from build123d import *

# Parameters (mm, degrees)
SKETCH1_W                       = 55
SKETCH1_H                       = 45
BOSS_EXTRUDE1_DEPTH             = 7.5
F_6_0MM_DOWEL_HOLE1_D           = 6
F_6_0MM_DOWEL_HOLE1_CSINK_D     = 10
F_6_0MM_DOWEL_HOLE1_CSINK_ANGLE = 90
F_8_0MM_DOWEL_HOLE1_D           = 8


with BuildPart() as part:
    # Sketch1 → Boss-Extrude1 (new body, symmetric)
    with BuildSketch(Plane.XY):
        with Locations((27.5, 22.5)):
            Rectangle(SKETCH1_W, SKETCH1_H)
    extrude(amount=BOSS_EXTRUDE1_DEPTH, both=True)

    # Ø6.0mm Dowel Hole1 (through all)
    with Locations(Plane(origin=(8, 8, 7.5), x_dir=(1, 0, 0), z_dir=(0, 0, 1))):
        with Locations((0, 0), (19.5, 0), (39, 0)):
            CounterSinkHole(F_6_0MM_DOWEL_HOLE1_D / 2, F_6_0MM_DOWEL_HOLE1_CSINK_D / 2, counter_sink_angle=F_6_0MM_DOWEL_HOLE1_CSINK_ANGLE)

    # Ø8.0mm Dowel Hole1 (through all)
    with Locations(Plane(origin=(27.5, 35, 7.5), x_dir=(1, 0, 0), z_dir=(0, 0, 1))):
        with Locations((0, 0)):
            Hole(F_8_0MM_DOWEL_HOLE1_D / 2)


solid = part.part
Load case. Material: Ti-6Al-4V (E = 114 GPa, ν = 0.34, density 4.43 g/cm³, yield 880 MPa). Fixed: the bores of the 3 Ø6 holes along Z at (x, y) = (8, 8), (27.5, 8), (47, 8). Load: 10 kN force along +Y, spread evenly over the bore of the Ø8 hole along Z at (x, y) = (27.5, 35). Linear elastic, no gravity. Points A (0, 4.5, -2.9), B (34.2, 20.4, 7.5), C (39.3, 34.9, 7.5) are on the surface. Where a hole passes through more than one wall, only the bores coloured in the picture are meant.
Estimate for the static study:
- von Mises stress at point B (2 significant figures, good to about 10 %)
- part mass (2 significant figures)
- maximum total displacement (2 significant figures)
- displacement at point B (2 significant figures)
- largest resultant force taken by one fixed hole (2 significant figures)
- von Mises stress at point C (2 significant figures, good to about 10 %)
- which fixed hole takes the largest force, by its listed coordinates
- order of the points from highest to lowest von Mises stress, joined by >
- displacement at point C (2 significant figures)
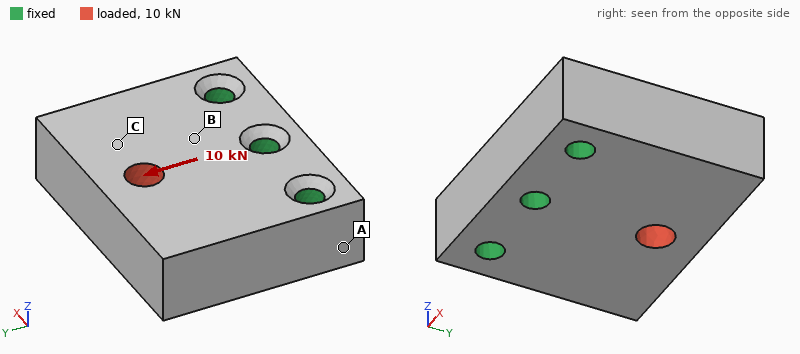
19 MPa
150 g
8.4 µm
2.4 µm
4.3 kN
11 MPa
(27.5, 8)
B > C > A
3.4 µm
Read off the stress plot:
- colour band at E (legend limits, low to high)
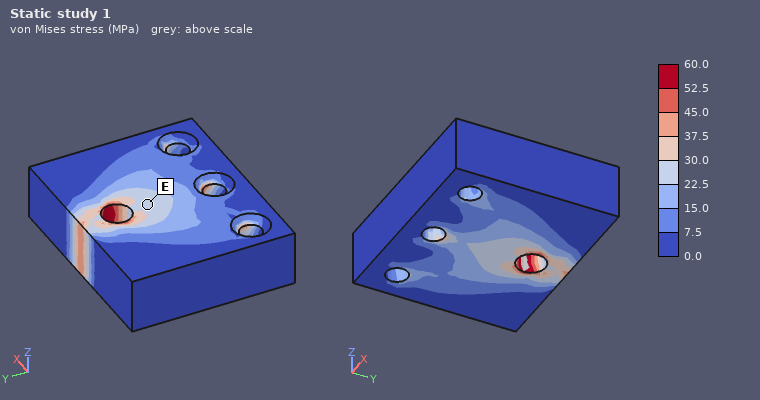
22.5 to 30.0 MPa
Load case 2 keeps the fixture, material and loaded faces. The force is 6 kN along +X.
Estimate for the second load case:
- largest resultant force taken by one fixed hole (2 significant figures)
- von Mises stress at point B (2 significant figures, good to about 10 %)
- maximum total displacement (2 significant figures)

4.1 kN
17 MPa
9.5 µm
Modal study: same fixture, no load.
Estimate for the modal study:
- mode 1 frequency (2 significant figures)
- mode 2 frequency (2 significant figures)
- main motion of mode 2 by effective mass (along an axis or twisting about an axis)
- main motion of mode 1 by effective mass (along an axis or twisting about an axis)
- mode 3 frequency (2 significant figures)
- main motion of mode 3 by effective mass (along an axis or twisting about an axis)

7900 Hz
12 kHz
twisting about Y
along Z
16 kHz
along X
